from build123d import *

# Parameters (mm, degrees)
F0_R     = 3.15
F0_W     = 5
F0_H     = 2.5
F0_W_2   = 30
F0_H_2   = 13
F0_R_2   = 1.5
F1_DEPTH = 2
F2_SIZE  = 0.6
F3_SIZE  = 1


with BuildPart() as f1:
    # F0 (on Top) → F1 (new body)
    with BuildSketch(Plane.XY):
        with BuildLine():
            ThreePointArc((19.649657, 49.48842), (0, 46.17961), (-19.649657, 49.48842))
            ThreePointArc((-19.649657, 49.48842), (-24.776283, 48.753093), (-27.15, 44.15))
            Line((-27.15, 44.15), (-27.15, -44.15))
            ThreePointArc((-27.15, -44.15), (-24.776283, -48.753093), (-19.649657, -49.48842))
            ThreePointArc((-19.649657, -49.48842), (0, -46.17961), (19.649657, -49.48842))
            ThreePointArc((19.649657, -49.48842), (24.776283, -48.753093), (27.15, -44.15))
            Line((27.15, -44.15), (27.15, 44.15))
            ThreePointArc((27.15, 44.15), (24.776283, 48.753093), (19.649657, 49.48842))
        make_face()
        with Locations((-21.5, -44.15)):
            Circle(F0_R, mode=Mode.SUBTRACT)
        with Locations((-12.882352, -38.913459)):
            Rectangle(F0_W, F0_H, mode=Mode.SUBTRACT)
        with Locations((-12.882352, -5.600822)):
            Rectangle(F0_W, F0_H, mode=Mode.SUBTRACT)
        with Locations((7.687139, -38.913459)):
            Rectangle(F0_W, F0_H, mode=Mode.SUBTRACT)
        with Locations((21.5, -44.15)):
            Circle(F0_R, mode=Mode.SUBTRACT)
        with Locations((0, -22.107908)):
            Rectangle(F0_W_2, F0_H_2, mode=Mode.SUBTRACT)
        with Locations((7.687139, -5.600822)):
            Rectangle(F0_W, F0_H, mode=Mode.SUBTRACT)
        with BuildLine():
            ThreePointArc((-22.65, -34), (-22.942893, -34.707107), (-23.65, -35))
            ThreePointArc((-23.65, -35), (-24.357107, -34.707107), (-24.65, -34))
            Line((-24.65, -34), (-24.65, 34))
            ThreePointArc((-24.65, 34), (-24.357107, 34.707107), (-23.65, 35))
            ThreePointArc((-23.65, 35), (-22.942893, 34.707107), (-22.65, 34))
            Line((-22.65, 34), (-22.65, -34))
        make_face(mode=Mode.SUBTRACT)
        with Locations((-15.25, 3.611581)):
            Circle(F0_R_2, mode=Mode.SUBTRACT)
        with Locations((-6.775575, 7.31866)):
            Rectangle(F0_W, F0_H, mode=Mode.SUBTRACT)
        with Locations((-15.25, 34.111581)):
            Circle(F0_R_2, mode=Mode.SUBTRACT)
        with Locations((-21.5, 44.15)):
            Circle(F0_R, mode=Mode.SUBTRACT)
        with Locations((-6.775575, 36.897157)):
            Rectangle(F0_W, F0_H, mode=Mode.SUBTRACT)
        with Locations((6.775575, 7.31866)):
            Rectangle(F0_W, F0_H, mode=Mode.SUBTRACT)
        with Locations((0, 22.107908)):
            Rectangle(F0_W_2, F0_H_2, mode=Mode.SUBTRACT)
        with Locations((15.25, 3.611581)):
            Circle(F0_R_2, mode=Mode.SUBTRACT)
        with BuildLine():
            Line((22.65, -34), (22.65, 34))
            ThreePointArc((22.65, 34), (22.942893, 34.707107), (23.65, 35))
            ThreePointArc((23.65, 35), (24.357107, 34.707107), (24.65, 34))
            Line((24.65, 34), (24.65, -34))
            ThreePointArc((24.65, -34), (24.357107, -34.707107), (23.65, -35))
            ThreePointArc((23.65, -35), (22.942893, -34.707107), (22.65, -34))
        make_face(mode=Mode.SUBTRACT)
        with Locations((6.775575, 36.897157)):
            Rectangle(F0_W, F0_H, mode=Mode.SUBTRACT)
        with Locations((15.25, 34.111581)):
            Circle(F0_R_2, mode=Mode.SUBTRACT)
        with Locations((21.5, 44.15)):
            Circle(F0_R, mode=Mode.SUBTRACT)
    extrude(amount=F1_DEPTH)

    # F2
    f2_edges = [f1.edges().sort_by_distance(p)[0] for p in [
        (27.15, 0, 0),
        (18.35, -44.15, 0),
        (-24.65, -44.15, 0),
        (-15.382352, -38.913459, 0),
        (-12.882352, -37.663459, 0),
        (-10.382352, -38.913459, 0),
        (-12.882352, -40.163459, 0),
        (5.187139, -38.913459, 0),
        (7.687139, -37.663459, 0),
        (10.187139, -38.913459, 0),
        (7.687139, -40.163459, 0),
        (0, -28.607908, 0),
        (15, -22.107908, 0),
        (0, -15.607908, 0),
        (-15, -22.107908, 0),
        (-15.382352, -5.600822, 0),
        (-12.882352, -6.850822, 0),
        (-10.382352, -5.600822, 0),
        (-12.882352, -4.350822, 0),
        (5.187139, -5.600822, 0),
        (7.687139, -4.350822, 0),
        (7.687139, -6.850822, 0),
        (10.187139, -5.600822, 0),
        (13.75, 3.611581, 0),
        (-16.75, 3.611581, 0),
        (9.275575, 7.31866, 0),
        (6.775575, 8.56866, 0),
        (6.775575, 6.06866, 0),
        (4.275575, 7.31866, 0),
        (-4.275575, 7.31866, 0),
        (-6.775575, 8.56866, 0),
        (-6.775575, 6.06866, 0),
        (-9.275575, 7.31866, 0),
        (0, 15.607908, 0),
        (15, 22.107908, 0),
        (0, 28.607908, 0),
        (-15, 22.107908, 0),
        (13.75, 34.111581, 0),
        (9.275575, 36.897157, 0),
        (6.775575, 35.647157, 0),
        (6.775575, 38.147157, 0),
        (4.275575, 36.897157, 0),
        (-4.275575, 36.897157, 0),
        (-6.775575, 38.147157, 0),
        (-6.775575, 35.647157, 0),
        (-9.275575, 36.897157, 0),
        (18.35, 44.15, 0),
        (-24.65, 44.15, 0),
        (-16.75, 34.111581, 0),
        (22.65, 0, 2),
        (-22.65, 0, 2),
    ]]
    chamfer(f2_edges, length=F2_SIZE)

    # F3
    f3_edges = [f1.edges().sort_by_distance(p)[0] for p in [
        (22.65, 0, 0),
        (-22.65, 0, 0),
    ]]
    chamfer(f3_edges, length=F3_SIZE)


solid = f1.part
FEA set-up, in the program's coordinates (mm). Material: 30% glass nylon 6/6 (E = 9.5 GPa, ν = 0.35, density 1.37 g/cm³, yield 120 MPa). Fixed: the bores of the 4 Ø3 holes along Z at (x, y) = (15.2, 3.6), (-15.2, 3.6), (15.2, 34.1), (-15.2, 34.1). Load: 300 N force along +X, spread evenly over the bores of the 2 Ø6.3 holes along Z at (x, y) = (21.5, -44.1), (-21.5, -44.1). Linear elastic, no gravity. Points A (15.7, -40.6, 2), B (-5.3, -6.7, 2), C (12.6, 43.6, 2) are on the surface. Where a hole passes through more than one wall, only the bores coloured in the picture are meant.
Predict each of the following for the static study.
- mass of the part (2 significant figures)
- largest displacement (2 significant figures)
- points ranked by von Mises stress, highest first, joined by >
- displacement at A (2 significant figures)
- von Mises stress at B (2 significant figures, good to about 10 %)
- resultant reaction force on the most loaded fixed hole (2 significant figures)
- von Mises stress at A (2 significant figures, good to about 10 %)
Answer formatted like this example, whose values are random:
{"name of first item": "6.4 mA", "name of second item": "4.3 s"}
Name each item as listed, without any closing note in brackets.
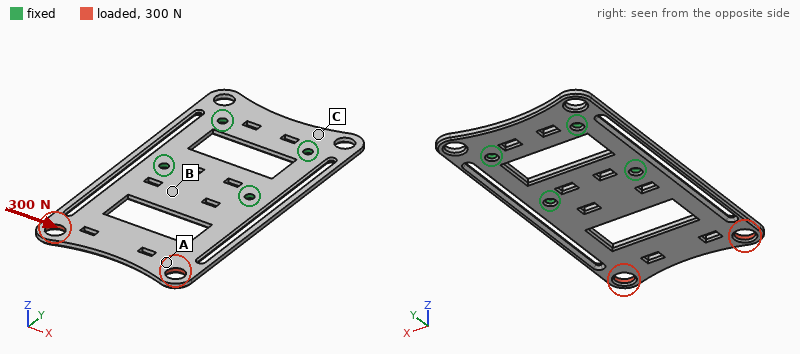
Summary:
{"mass of the part": "10 g", "largest displacement": "0.58 mm", "points ranked by von Mises stress, highest first, joined by >": "B > A > C", "displacement at A": "0.45 mm", "von Mises stress at B": "19 MPa", "resultant reaction force on the most loaded fixed hole": "380 N", "von Mises stress at A": "9.7 MPa"}
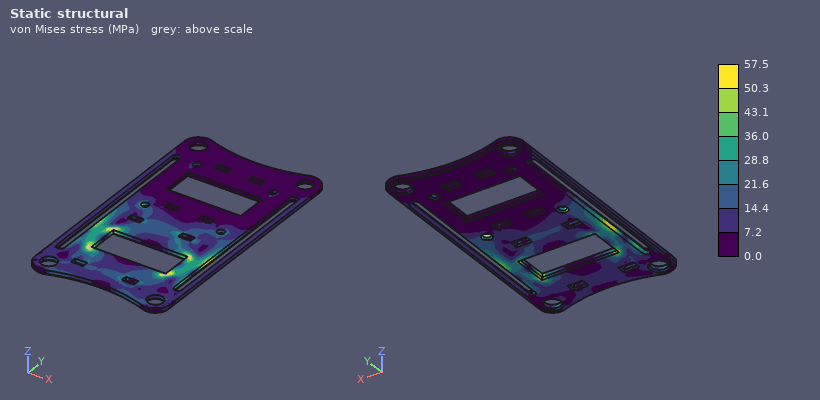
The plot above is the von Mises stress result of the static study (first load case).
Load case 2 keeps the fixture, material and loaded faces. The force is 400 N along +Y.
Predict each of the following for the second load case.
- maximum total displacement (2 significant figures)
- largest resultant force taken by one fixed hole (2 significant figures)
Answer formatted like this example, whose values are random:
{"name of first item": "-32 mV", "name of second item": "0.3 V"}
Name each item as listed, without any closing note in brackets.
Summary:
{"maximum total displacement": "0.97 mm", "largest resultant force taken by one fixed hole": "170 N"}
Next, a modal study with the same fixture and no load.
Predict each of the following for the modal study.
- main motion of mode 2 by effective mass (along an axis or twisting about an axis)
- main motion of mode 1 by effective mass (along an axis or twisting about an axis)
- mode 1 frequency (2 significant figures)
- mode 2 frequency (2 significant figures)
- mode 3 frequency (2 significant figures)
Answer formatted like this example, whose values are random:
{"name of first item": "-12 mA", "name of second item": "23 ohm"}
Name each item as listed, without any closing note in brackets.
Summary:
{"main motion of mode 2 by effective mass": "twisting about Y", "main motion of mode 1 by effective mass": "along Z", "mode 1 frequency": "260 Hz", "mode 2 frequency": "580 Hz", "mode 3 frequency": "810 Hz"}
